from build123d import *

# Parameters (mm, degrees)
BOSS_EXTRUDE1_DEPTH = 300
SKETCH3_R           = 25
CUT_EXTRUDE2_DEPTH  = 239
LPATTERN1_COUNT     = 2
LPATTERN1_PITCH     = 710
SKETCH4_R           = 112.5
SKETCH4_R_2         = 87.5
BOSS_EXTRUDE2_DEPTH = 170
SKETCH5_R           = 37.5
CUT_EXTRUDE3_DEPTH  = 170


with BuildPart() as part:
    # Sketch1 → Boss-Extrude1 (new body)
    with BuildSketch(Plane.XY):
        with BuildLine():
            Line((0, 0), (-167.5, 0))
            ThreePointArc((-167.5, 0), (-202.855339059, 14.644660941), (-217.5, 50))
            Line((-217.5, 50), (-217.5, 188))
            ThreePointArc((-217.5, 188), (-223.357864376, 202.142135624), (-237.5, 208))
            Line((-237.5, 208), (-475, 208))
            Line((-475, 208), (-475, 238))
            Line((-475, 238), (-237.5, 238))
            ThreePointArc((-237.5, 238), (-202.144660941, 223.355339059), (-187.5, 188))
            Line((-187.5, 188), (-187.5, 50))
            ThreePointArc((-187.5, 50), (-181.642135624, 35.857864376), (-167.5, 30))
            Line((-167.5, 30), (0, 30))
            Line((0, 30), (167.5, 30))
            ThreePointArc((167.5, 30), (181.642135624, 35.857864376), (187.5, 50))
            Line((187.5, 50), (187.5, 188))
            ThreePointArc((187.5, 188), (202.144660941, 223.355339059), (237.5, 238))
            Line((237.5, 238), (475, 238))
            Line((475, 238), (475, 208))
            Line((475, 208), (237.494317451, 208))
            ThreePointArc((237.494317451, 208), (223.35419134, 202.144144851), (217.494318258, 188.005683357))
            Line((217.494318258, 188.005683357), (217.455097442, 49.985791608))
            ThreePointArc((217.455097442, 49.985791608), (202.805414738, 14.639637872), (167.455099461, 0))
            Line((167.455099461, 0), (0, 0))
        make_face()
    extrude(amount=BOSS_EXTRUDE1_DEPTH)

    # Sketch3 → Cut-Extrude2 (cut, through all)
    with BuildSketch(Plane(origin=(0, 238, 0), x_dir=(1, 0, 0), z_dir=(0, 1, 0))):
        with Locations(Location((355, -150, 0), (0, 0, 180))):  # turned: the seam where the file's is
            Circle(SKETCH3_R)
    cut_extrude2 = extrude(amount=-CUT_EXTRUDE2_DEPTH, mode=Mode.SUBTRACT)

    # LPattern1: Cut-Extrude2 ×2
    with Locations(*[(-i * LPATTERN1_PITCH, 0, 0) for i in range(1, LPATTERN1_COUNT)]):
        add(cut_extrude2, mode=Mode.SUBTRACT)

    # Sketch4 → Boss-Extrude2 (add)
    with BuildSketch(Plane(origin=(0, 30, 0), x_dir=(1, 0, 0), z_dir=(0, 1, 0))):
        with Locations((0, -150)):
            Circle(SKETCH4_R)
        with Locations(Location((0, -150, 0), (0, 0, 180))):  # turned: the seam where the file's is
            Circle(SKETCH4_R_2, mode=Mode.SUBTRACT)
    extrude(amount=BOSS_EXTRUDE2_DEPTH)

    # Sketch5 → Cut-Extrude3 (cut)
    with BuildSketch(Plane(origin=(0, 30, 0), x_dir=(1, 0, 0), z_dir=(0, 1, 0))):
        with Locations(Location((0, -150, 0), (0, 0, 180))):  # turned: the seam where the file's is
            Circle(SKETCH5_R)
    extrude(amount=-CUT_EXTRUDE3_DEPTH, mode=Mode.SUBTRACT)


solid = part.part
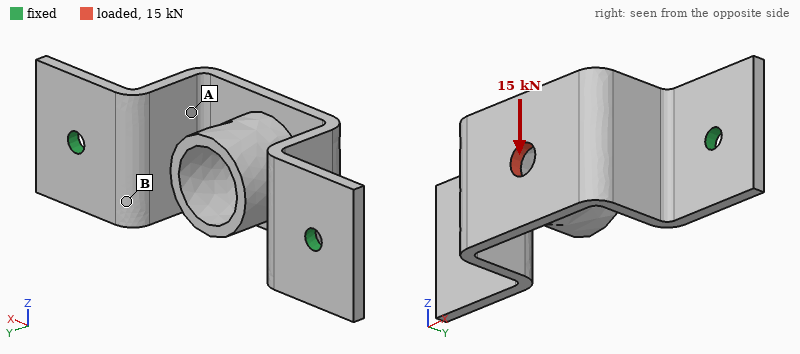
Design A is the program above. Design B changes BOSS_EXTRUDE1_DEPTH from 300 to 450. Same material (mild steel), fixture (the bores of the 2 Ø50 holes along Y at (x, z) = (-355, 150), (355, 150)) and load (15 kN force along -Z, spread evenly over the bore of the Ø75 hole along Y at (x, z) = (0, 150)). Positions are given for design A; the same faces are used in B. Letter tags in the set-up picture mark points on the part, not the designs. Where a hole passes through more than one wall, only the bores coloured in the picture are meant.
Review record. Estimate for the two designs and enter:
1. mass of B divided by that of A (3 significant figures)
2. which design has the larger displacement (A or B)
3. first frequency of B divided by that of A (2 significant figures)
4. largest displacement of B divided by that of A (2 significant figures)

1.41
B
0.75
1.2
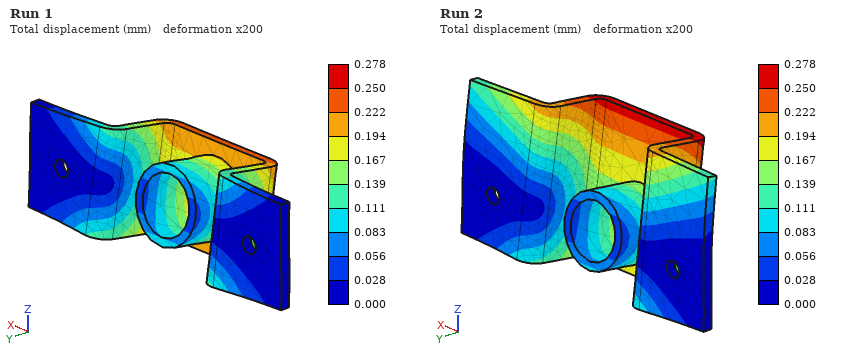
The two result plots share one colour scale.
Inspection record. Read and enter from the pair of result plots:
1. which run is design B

Run 2
